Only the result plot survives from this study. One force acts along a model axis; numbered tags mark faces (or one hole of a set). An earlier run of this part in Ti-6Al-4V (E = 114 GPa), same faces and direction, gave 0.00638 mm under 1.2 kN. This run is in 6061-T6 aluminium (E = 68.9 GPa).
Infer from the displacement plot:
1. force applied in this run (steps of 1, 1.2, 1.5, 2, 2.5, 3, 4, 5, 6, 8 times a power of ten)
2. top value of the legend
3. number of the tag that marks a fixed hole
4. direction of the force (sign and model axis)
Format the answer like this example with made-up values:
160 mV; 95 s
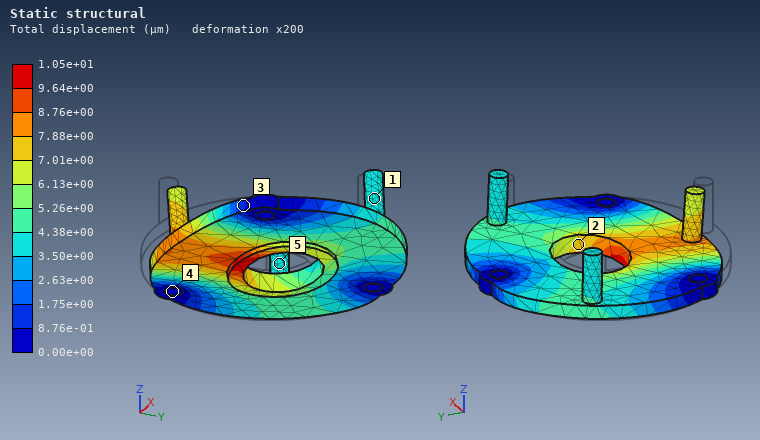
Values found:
1.2 kN; 1.05e+01 µm; 4; +Y
